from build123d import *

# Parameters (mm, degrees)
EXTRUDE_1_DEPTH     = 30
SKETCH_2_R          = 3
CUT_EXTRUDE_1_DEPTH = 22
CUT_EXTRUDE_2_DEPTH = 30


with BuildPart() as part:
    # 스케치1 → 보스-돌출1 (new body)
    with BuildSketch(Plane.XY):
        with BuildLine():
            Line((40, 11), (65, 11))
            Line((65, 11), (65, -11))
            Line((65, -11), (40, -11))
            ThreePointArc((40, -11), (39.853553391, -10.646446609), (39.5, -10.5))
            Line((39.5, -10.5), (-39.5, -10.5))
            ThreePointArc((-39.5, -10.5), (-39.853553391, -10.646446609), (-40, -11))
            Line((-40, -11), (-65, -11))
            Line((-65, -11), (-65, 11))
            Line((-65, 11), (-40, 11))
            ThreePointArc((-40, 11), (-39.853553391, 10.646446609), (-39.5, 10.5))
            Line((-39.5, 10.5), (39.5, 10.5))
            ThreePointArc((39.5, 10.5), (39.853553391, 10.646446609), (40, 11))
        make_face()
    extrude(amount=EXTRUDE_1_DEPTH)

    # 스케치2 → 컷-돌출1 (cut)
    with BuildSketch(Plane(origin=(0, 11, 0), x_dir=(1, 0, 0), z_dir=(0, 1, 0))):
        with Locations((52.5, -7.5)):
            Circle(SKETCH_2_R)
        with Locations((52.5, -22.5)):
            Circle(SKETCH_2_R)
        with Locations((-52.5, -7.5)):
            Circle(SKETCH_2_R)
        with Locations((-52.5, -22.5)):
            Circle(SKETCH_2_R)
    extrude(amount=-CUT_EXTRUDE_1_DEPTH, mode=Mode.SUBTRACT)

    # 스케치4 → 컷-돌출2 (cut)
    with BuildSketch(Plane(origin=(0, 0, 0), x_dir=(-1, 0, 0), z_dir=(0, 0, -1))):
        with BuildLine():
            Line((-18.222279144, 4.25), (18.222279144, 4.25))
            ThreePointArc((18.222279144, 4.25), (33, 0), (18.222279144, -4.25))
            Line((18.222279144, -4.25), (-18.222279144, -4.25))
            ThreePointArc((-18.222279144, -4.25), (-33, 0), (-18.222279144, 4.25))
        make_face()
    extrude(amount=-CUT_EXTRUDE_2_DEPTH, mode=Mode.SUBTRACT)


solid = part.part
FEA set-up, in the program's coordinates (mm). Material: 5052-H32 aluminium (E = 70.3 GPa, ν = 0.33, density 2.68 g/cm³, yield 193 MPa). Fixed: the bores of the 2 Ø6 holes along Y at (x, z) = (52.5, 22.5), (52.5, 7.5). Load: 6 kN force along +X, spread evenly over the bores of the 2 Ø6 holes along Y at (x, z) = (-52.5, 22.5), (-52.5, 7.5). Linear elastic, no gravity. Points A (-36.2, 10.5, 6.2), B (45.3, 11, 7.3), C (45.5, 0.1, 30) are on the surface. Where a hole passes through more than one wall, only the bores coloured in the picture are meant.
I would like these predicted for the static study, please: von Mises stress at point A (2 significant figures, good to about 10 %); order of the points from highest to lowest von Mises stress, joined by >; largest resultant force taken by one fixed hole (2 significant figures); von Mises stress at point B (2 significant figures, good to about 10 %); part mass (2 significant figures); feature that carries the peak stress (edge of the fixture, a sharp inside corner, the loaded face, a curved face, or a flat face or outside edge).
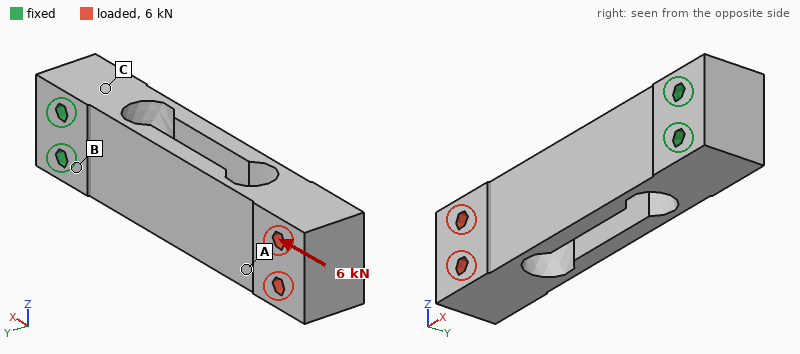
26 MPa
A > B > C
3.0 kN
13 MPa
160 g
a curved face
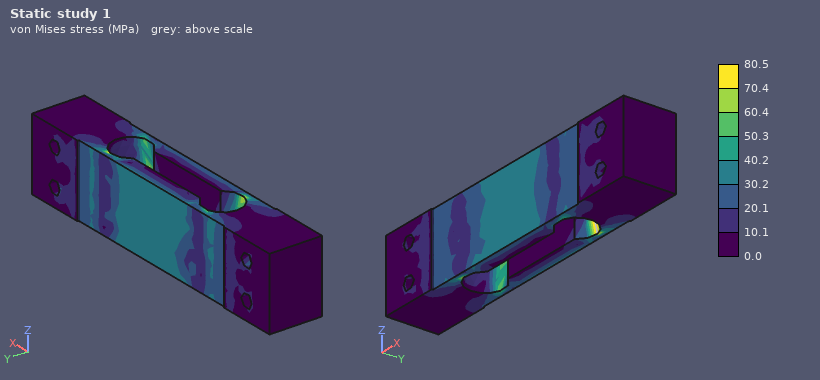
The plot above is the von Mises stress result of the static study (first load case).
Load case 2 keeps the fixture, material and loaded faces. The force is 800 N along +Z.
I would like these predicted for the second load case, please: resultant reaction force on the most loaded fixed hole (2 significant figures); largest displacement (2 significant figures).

4.5 kN
0.25 mm
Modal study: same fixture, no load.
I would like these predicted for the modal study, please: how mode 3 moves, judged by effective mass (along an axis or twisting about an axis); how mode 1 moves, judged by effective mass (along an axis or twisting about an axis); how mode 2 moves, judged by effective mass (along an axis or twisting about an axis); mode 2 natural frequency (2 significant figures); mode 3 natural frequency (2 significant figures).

twisting about X
along Y
along Z
1300 Hz
2600 Hz
